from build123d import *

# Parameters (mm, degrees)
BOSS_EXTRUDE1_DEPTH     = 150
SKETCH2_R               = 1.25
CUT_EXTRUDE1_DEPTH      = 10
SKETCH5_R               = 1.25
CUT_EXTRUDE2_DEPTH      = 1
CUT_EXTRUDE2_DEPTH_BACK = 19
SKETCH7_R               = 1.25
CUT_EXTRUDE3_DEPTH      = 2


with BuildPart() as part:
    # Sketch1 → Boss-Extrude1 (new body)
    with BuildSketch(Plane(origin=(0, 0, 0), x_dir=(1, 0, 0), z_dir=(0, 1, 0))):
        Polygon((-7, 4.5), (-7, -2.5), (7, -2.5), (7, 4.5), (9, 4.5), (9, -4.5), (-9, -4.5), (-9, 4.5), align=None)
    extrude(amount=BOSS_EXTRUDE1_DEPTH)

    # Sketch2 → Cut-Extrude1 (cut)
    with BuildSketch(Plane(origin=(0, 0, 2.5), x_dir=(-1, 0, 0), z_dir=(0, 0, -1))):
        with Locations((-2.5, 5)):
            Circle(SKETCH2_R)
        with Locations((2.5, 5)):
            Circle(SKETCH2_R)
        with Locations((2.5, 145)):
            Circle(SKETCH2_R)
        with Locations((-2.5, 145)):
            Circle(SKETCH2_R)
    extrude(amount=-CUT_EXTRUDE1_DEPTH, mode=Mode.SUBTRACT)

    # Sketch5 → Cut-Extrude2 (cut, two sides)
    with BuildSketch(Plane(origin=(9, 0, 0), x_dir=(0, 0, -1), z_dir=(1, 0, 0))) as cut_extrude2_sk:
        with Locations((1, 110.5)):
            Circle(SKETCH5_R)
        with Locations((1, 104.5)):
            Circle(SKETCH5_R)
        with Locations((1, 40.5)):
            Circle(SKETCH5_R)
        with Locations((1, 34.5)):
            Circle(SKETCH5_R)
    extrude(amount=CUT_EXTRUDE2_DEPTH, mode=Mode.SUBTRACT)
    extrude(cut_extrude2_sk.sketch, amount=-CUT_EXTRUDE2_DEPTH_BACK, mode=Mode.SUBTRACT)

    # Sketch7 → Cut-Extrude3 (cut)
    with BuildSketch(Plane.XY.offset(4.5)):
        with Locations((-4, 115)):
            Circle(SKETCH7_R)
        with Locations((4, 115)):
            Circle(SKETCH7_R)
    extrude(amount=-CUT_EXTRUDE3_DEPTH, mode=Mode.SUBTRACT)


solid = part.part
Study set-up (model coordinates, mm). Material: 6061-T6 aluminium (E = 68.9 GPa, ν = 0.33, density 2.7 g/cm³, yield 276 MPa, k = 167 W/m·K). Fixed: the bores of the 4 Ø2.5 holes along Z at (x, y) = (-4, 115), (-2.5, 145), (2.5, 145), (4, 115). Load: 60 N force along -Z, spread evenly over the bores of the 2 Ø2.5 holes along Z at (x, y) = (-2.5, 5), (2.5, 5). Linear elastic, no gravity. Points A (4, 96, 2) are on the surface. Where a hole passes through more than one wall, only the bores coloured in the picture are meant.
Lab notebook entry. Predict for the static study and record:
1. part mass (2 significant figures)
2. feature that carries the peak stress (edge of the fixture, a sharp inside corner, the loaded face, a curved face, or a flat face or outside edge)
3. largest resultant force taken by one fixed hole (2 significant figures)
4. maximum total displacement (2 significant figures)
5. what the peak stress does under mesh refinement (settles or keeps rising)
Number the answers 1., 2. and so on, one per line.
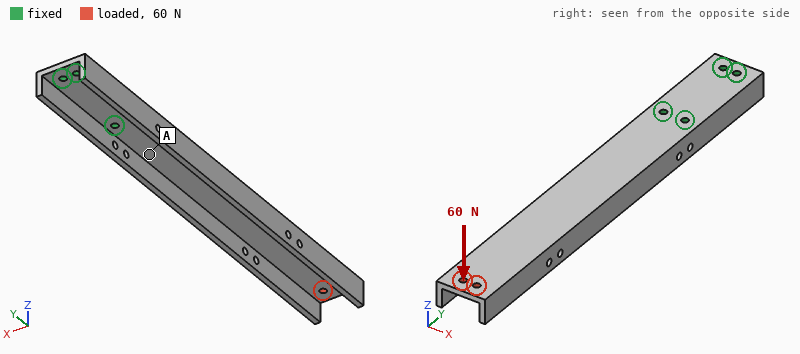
1. 26 g
2. edge of the fixture
3. 230 N
4. 1.2 mm
5. keeps rising
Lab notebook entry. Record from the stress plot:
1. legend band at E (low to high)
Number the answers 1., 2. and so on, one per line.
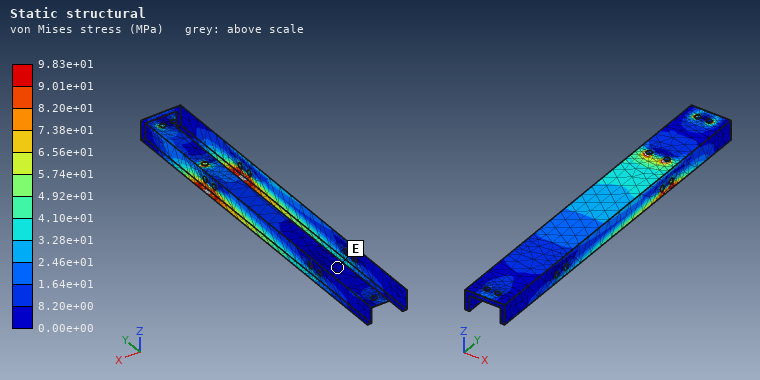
1. 0.00e+00 to 8.20e+00 MPa
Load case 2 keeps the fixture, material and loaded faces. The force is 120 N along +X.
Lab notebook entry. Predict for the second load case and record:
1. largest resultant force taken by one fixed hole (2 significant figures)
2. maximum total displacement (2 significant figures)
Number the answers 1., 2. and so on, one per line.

1. 790 N
2. 0.52 mm
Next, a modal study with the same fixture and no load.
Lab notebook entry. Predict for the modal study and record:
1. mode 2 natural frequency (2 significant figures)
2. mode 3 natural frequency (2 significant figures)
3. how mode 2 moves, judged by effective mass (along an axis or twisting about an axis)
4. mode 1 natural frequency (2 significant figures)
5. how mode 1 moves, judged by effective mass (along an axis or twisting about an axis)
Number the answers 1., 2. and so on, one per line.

1. 960 Hz
2. 1600 Hz
3. along X
4. 490 Hz
5. along Z
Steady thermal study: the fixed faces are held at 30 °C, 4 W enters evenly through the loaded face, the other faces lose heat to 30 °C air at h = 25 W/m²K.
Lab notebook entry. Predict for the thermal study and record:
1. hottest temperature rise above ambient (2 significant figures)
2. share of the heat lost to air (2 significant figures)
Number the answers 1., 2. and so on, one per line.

1. 28 K
2. 58 %
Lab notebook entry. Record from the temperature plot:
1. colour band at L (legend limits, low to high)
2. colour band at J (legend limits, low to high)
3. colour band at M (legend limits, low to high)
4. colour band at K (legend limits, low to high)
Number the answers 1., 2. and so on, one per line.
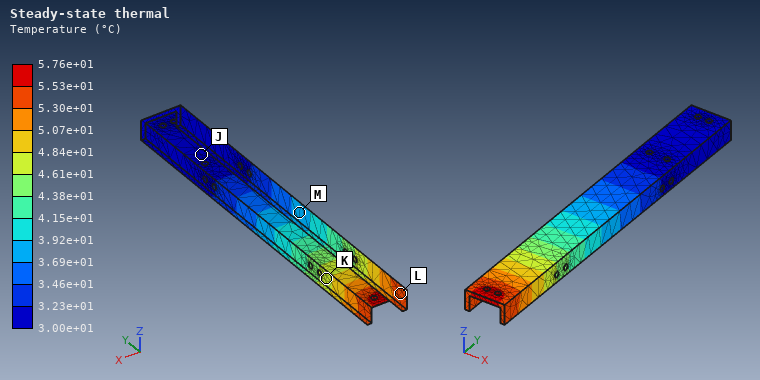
1. 5.30e+01 to 5.53e+01 °C
2. 3.00e+01 to 3.23e+01 °C
3. 3.69e+01 to 3.92e+01 °C
4. 4.61e+01 to 4.84e+01 °C
